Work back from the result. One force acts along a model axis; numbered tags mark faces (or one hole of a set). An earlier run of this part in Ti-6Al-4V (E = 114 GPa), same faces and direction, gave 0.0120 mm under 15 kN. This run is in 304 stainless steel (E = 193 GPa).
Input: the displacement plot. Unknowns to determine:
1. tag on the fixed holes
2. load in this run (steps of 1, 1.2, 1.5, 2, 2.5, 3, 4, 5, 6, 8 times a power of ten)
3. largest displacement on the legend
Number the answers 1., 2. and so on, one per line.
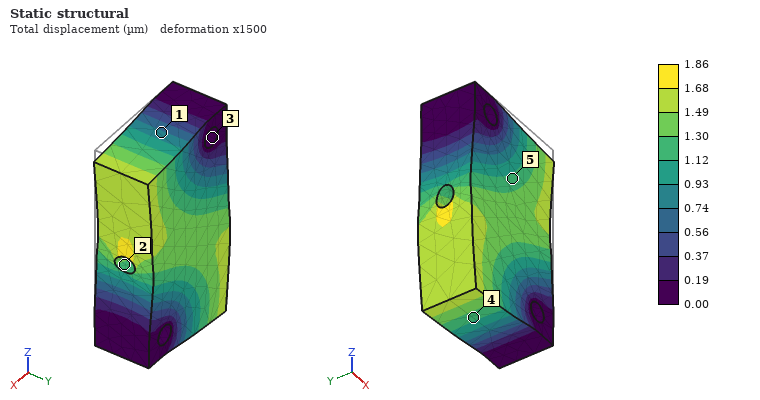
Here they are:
1. 3
2. 4 kN
3. 1.86 µm
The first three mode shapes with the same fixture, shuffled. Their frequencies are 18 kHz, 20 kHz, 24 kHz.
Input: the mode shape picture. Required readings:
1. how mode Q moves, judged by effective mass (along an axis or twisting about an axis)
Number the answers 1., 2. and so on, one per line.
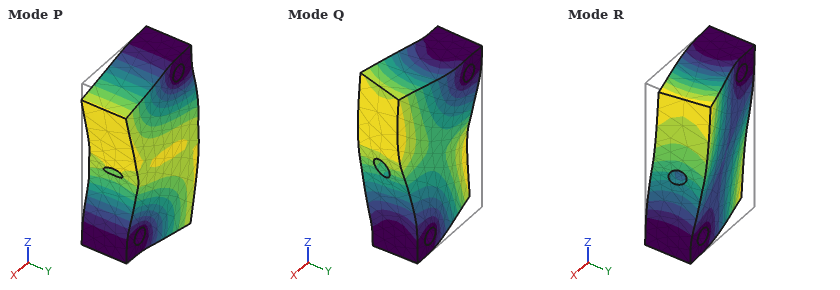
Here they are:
1. along Y
